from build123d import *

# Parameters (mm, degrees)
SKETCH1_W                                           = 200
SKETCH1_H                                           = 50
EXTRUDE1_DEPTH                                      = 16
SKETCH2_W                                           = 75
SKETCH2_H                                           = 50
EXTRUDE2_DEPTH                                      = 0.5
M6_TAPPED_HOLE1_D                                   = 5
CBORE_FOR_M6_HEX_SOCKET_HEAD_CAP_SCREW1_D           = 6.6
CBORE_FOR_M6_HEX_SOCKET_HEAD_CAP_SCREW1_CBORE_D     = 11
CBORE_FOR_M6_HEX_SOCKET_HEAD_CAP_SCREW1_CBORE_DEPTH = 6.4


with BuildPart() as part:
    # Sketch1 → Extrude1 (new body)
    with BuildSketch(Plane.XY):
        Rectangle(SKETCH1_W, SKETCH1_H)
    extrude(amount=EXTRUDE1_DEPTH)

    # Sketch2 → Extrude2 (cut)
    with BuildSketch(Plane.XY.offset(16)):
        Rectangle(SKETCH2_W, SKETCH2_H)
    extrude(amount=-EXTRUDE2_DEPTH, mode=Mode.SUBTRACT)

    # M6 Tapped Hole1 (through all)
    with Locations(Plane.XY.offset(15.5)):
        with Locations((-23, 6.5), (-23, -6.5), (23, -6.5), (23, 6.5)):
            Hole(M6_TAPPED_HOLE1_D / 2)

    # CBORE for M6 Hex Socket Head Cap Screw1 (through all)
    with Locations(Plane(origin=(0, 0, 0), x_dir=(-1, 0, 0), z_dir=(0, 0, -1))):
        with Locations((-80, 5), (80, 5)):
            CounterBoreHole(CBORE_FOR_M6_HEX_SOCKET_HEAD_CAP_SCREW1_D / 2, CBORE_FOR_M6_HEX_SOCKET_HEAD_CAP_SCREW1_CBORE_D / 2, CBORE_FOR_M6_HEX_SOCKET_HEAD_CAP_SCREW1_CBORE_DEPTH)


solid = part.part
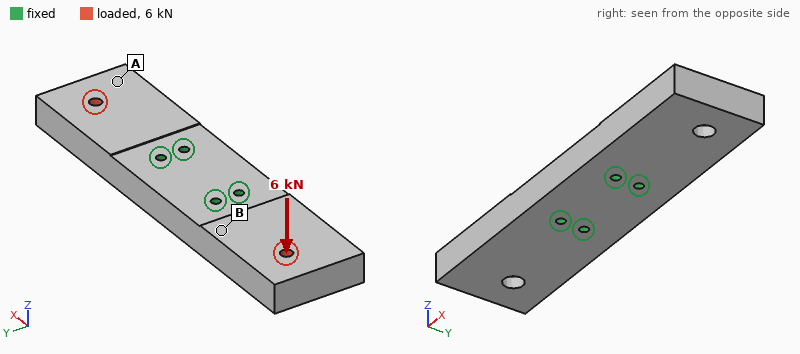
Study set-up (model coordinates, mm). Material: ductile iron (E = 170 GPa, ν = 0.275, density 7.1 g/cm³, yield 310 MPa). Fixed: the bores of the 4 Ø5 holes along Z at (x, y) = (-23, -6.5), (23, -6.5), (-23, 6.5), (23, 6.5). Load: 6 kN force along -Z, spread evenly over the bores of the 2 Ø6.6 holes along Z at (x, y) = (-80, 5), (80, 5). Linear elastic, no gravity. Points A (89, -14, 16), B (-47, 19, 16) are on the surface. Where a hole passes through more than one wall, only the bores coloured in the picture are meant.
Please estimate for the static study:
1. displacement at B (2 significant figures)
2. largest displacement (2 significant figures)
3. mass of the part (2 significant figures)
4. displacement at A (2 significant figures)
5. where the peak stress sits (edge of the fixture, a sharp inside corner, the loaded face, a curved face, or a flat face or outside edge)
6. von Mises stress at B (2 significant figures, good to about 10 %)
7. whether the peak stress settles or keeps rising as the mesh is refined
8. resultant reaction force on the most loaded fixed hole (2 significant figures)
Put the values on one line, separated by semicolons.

0.025 mm; 0.12 mm; 1.1 kg; 0.094 mm; edge of the fixture; 46 MPa; keeps rising; 2.0 kN
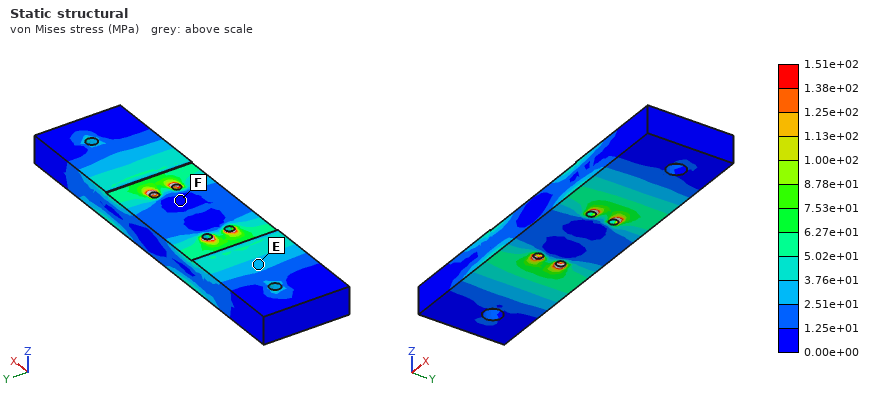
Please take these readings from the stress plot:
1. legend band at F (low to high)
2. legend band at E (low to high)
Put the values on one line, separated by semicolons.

0.00e+00 to 1.25e+01 MPa; 2.51e+01 to 3.76e+01 MPa
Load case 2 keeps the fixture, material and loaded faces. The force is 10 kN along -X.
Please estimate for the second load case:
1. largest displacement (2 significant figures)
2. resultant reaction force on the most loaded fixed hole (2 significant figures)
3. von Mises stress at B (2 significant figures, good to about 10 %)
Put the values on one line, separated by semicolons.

19 µm; 3.3 kN; 16 MPa
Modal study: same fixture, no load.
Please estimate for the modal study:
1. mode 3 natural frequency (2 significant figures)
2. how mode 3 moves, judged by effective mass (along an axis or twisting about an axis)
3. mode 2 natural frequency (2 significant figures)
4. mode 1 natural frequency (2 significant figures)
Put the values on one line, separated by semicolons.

4000 Hz; twisting about Z; 2000 Hz; 1900 Hz
